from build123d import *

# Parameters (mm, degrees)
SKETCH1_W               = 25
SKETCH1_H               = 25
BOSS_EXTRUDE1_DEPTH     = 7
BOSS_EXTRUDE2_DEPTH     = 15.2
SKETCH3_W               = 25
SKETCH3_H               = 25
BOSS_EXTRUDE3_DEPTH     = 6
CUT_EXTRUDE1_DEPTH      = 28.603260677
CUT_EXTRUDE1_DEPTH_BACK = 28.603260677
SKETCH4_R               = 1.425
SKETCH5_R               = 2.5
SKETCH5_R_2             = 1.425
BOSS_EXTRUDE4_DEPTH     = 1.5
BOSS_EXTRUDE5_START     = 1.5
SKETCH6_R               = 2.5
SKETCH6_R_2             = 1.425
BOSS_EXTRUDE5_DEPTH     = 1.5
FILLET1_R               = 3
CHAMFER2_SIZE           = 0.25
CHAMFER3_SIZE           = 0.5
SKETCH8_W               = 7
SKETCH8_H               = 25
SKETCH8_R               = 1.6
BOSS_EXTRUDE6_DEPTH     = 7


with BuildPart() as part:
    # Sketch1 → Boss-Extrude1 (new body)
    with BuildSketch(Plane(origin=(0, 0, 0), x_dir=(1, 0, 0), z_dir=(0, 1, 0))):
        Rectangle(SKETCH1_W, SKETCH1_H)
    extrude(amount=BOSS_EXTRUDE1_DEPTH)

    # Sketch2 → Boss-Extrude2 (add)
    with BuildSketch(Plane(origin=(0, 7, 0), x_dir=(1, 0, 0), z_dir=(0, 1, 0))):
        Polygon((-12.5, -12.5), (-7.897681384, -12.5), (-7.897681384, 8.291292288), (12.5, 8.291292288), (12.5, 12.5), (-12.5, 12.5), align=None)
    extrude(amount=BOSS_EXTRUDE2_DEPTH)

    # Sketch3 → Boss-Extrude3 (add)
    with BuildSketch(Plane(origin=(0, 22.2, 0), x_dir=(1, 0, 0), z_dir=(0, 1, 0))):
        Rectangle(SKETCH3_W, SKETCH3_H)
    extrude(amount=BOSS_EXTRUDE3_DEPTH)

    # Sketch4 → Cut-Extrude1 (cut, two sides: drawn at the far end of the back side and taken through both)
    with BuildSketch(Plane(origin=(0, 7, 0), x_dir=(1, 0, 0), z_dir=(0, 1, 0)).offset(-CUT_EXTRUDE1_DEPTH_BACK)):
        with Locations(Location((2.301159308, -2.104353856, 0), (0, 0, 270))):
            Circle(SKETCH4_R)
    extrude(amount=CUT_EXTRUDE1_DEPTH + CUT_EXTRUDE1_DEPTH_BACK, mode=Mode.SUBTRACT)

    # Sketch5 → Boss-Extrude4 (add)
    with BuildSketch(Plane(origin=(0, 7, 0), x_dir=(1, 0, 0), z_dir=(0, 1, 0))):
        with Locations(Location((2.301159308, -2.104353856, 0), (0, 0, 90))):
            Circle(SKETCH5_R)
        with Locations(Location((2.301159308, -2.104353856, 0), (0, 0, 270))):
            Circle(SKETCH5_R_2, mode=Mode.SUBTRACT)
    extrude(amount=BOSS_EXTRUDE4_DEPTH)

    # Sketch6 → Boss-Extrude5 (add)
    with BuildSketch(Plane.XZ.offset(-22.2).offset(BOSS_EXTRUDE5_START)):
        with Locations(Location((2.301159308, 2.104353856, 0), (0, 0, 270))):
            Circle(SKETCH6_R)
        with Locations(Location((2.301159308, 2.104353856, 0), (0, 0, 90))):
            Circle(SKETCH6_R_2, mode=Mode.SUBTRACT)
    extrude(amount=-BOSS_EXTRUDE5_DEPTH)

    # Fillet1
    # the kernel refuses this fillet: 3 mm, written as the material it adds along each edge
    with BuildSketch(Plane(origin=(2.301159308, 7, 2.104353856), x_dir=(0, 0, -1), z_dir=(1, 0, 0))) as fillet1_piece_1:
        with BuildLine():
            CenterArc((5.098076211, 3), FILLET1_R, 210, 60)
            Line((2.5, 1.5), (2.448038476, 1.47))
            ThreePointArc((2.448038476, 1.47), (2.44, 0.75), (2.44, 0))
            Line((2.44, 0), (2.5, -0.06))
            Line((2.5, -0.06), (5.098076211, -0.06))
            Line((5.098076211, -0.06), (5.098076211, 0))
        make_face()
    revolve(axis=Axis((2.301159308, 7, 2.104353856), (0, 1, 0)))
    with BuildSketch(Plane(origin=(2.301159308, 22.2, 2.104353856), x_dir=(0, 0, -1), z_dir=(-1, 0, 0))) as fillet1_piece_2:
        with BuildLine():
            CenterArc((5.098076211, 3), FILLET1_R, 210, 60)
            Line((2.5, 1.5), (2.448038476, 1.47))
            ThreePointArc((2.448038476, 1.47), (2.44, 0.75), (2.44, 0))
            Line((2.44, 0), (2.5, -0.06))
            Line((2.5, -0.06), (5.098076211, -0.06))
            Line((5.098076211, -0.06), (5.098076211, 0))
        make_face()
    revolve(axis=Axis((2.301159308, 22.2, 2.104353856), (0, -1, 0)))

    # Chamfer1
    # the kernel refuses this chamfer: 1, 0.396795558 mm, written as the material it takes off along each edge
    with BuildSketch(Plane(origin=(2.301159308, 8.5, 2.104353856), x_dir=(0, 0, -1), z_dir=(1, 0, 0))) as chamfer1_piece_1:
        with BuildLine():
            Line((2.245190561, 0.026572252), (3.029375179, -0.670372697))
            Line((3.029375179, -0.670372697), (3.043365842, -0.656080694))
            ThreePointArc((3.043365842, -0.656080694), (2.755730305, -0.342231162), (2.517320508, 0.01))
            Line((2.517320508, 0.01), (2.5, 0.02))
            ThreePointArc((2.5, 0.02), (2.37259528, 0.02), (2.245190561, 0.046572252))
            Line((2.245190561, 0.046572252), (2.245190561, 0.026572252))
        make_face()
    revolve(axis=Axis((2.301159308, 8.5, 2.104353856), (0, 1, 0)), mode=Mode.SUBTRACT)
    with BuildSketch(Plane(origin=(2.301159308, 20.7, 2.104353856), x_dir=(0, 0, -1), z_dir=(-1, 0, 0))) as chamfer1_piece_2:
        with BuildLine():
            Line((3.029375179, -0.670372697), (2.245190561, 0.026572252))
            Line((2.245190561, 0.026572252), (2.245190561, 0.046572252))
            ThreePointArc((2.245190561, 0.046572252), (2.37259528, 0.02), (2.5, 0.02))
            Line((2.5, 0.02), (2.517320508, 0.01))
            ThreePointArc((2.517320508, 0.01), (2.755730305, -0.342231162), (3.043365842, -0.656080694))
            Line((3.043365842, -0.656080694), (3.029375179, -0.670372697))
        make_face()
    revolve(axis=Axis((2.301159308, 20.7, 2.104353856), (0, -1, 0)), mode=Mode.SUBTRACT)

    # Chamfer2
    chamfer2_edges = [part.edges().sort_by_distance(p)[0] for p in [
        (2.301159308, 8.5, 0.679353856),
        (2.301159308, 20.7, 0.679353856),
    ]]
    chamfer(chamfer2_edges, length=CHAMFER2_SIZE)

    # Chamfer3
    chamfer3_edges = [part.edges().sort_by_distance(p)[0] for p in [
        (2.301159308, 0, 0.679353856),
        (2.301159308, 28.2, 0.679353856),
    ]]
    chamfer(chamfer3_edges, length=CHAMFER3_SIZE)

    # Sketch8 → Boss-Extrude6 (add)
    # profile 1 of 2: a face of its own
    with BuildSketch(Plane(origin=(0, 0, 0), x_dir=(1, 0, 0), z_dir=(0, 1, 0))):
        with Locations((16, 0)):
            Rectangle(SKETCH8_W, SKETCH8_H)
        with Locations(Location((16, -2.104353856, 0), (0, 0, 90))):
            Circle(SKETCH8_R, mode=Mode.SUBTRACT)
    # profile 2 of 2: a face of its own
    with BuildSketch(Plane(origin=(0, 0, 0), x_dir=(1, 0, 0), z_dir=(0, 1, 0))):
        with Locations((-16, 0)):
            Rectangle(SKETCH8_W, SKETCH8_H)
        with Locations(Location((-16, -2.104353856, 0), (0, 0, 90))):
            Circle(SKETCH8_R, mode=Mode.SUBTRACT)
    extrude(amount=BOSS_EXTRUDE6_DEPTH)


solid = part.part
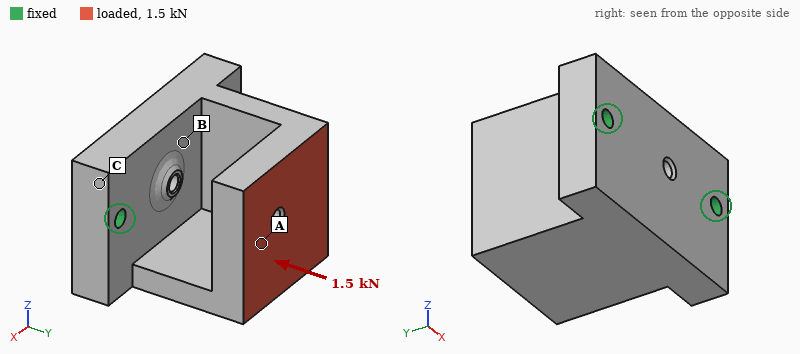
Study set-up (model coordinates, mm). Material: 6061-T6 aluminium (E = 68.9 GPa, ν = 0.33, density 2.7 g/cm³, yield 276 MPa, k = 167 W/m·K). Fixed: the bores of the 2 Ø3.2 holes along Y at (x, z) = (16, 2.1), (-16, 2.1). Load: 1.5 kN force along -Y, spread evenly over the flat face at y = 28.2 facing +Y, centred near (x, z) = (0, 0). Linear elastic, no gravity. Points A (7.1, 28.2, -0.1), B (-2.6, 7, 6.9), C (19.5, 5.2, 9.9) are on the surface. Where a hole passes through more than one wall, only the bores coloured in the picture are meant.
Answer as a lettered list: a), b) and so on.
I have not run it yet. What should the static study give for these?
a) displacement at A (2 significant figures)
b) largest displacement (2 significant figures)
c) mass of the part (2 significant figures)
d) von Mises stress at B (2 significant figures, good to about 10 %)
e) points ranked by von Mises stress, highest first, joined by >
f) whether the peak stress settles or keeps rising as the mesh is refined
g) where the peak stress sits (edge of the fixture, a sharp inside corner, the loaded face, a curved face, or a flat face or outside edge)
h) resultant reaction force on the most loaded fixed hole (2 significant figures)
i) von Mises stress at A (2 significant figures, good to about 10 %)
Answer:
a) 50 µm
b) 89 µm
c) 36 g
d) 15 MPa
e) A > B > C
f) keeps rising
g) edge of the fixture
h) 780 N
i) 26 MPa
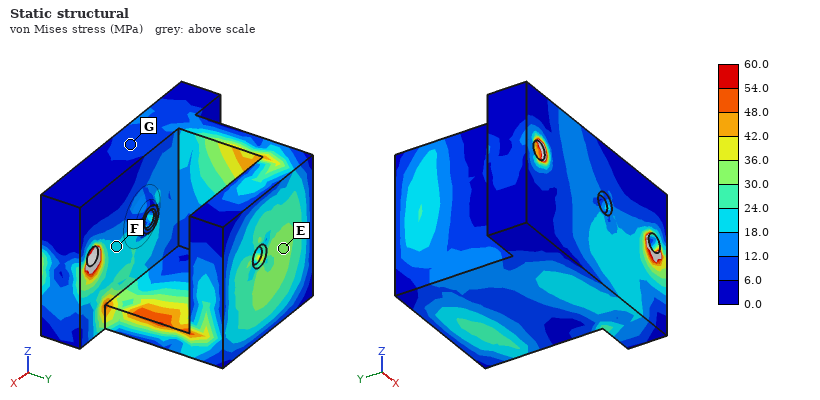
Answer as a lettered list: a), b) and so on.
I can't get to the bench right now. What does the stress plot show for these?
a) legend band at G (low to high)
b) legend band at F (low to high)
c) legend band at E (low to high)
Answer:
a) 6.0 to 12.0 MPa
b) 18.0 to 24.0 MPa
c) 30.0 to 36.0 MPa
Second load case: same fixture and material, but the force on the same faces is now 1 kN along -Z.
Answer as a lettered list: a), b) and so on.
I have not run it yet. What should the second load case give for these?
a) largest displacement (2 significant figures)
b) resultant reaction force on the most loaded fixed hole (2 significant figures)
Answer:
a) 0.13 mm
b) 530 N
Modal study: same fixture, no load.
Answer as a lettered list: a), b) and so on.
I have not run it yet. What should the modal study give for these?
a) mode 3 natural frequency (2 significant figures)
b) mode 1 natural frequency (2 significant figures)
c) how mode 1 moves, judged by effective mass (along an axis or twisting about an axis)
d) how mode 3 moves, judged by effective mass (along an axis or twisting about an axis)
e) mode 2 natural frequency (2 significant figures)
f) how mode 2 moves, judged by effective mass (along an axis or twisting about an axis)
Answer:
a) 10 kHz
b) 4900 Hz
c) along Z
d) along Y
e) 5900 Hz
f) along X
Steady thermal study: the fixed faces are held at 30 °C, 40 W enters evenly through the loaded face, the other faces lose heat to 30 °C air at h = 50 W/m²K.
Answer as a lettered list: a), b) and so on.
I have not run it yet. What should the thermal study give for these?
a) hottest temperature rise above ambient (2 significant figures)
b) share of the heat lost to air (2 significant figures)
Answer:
a) 39 K
b) 9.8 %
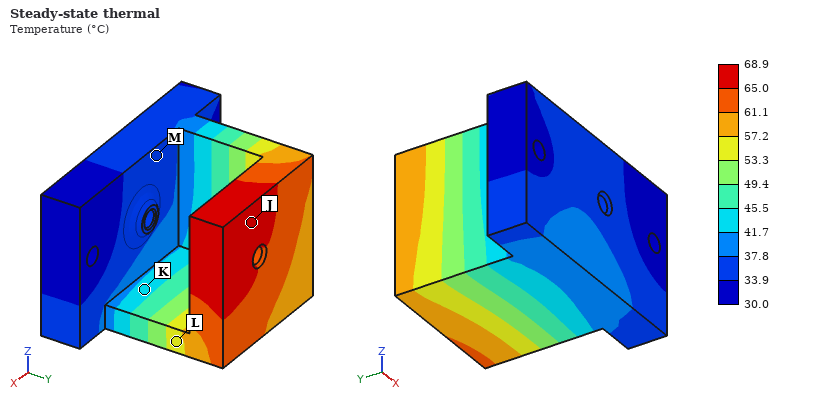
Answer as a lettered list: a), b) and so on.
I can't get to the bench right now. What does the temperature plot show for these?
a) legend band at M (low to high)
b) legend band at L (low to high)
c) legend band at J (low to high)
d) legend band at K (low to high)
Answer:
a) 33.9 to 37.8 °C
b) 53.3 to 57.2 °C
c) 65.0 to 68.9 °C
d) 41.7 to 45.5 °C
